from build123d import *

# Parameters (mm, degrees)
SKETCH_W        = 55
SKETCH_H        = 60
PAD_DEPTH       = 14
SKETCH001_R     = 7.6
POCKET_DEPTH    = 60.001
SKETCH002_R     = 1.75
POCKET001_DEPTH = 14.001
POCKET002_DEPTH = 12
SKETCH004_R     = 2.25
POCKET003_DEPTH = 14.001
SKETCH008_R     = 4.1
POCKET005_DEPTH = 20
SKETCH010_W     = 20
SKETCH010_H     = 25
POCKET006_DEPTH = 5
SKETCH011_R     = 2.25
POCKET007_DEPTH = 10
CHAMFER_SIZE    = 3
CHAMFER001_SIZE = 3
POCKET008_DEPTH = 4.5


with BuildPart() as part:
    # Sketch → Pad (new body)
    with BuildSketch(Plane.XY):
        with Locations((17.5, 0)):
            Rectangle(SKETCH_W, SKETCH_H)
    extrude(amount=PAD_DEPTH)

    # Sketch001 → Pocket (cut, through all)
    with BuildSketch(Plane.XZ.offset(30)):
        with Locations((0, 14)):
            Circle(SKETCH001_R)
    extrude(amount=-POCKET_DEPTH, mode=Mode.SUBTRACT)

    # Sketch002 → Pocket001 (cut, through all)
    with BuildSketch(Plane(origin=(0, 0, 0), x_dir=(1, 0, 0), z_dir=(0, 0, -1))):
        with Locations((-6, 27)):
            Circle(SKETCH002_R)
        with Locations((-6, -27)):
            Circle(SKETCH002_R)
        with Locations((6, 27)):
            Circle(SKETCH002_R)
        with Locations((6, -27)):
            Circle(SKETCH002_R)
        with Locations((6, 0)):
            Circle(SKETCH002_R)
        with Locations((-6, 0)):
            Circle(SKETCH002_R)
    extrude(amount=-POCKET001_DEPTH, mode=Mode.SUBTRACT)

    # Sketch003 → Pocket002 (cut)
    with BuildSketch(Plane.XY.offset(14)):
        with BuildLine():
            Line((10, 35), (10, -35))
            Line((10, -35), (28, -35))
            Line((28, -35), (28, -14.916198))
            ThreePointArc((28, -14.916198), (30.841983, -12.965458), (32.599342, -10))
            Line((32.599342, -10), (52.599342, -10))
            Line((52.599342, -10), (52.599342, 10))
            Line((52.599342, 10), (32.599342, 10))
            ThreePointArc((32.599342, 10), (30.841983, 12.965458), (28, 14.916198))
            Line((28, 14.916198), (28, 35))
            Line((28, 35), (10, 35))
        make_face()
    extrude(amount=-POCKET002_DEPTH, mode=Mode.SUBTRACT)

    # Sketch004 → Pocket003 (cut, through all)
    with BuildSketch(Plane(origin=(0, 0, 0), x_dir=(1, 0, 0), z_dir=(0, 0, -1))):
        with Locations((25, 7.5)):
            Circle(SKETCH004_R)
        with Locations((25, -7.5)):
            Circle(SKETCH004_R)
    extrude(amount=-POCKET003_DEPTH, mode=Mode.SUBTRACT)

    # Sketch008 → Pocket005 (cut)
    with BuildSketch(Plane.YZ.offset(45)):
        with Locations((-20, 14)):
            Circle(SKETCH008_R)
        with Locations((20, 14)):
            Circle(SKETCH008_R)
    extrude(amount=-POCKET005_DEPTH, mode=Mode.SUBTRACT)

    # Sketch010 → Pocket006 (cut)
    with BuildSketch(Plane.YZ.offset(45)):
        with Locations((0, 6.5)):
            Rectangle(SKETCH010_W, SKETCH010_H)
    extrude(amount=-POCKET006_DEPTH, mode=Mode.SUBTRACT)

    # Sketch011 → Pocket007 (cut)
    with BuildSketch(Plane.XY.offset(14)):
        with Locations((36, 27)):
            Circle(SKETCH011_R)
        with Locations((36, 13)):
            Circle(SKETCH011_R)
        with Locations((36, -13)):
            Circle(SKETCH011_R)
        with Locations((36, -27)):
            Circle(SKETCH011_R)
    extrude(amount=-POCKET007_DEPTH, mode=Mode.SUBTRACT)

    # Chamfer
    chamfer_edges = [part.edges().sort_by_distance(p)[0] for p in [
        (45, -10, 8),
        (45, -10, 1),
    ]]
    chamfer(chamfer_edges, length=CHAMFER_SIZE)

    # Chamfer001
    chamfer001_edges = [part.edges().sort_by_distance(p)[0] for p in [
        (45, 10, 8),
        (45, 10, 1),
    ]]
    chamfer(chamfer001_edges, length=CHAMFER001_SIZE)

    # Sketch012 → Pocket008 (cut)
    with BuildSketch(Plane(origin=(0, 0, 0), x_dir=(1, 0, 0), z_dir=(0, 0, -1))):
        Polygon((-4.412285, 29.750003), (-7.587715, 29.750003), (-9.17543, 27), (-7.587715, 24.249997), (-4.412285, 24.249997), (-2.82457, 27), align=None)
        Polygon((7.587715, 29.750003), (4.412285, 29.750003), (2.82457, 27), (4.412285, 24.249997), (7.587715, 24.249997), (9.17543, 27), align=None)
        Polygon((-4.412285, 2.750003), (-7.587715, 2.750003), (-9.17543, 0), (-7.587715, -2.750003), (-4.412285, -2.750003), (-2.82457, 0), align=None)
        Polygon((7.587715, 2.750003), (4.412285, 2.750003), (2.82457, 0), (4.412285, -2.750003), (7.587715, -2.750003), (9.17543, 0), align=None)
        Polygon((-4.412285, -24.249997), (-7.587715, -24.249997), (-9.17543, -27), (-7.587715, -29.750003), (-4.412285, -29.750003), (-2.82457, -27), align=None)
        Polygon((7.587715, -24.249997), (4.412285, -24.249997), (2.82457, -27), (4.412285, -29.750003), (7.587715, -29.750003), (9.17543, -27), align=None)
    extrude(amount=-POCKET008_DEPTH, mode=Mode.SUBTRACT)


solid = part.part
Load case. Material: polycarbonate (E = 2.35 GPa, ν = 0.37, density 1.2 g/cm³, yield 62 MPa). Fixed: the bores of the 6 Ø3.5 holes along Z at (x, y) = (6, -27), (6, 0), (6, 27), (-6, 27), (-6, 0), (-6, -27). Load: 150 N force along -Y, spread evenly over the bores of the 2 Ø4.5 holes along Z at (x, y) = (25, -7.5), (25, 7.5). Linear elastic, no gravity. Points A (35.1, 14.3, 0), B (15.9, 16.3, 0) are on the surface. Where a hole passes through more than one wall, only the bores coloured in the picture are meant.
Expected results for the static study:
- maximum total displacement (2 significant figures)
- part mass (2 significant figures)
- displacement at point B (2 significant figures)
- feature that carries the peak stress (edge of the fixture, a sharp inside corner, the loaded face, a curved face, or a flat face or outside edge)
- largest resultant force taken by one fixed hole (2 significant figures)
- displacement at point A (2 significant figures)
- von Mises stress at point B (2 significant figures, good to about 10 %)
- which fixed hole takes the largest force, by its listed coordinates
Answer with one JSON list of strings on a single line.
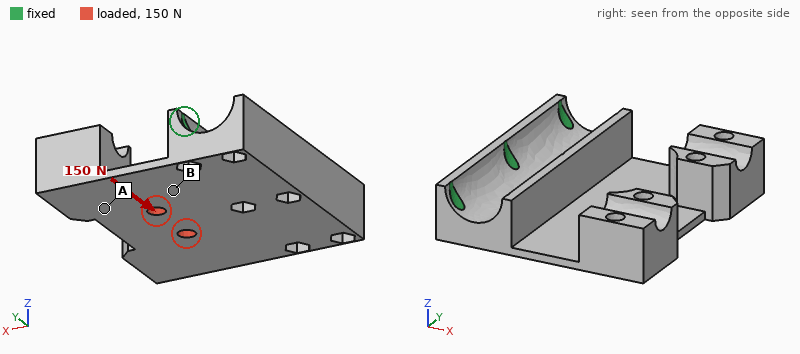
["93 µm", "25 g", "23 µm", "a flat face or outside edge", "68 N", "53 µm", "2.3 MPa", "(6, 0)"]
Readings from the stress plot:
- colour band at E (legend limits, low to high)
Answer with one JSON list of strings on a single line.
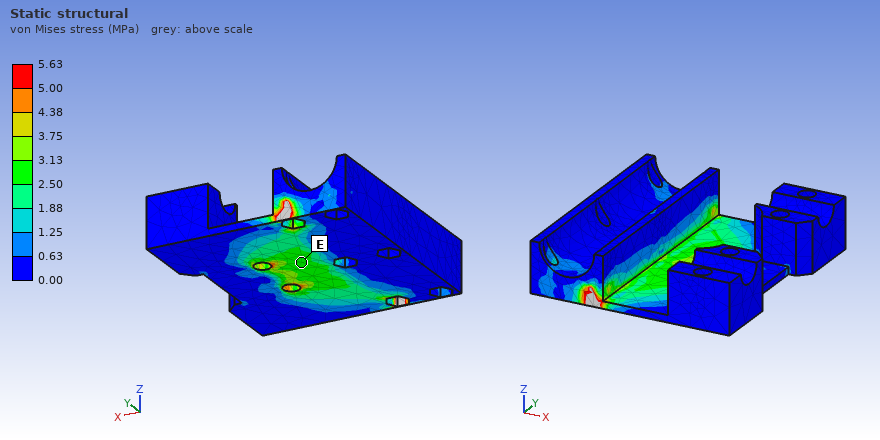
["2.50 to 3.13 MPa"]
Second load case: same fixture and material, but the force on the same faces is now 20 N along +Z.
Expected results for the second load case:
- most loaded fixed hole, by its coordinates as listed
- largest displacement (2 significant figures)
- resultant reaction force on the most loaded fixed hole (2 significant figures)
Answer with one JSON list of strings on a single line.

["(6, 0)", "0.86 mm", "28 N"]
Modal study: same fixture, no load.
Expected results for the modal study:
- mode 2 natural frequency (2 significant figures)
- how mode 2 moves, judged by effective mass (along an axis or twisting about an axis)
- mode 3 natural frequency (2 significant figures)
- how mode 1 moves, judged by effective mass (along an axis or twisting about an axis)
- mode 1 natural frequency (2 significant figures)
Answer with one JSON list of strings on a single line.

["280 Hz", "twisting about X", "690 Hz", "along Z", "180 Hz"]
